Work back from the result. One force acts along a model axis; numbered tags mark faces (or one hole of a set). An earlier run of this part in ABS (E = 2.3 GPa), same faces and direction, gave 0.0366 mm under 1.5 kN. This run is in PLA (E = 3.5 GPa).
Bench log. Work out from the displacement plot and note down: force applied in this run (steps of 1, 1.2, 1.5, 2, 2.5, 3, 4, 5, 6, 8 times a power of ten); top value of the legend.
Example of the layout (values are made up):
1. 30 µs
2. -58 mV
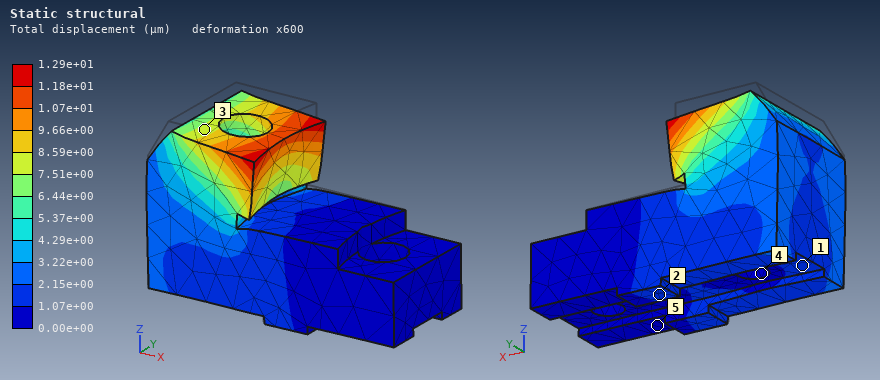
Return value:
1. 800 N
2. 1.29e+01 µm
